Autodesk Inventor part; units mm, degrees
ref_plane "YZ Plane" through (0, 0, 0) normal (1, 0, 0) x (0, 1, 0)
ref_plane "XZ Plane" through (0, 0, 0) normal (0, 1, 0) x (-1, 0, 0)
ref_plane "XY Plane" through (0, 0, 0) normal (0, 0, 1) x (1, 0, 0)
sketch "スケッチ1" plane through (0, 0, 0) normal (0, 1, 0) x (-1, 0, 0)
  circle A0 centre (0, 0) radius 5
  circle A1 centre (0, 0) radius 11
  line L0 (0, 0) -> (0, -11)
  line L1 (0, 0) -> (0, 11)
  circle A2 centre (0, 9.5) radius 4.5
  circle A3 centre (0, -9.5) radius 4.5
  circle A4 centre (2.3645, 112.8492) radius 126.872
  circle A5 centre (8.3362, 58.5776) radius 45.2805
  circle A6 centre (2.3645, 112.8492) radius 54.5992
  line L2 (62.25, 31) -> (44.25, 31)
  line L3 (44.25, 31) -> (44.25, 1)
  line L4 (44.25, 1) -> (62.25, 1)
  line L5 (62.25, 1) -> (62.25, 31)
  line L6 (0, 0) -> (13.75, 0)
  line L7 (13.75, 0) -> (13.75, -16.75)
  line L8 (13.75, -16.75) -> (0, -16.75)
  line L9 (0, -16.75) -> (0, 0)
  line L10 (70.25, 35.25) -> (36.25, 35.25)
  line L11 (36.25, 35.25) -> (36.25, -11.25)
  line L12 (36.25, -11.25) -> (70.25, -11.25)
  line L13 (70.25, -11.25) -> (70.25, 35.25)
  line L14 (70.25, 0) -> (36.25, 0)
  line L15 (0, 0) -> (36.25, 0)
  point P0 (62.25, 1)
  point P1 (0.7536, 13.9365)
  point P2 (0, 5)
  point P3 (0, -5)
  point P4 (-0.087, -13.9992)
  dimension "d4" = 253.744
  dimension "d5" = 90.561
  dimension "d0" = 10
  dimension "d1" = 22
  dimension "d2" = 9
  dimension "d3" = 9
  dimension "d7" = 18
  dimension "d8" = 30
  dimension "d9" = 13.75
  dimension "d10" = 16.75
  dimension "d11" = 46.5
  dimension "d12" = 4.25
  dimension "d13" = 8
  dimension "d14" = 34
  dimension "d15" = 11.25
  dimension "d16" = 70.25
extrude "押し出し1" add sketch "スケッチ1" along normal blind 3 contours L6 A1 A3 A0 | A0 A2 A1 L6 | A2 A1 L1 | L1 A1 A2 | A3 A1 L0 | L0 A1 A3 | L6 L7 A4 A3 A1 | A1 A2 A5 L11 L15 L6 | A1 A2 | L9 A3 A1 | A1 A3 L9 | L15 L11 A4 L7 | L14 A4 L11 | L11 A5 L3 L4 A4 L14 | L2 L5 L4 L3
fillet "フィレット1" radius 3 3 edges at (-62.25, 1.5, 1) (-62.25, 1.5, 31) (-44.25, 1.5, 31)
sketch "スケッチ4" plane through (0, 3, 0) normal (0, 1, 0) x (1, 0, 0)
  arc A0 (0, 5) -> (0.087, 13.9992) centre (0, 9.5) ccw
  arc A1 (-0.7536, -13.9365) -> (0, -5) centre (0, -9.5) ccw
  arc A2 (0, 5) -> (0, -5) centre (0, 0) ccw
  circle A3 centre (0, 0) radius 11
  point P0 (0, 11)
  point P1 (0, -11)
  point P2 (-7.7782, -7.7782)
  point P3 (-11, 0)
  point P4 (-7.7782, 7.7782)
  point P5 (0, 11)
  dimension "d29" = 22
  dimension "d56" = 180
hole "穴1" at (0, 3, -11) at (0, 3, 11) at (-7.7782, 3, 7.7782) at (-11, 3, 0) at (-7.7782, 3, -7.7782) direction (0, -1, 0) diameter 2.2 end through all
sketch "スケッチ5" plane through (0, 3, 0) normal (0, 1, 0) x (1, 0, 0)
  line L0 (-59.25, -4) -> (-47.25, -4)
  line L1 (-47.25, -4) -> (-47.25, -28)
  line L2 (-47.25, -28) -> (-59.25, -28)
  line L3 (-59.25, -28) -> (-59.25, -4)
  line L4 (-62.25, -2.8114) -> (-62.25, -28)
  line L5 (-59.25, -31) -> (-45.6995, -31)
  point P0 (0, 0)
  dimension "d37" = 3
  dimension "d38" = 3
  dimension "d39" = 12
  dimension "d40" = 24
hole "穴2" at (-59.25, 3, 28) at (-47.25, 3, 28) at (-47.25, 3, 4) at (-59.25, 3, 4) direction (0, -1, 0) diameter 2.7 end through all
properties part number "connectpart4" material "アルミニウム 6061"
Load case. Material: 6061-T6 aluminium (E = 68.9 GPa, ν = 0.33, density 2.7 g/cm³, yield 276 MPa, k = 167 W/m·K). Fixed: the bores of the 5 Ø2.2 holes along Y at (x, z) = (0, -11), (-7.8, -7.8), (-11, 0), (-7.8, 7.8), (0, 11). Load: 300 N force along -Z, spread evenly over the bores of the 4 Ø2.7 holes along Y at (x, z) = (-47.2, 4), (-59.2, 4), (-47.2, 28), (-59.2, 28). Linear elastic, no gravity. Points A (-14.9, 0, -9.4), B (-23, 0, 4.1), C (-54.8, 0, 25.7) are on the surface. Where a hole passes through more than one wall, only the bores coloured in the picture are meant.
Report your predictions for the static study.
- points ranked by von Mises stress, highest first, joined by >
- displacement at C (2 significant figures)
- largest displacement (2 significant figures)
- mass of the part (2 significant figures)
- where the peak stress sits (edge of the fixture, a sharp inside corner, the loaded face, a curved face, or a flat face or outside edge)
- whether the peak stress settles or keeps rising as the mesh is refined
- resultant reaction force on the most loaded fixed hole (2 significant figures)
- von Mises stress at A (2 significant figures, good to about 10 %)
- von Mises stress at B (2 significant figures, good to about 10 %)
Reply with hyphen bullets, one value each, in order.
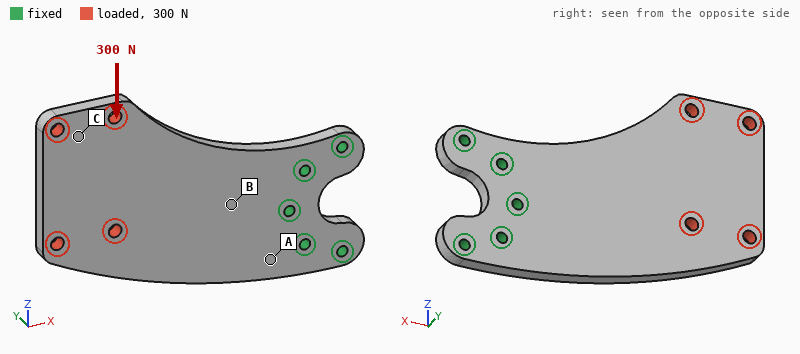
- A > B > C
- 46 µm
- 55 µm
- 15 g
- edge of the fixture
- keeps rising
- 530 N
- 24 MPa
- 10 MPa
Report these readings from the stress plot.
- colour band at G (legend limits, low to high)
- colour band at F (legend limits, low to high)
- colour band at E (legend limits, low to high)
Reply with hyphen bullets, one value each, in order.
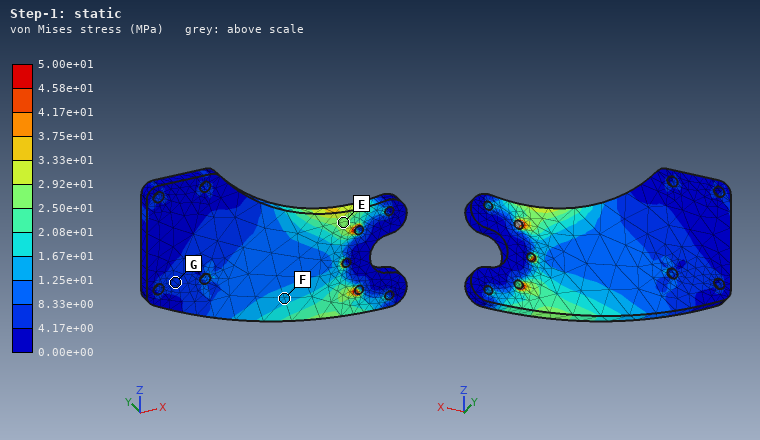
- 4.17e+00 to 8.33e+00 MPa
- 1.25e+01 to 1.67e+01 MPa
- 2.50e+01 to 2.92e+01 MPa
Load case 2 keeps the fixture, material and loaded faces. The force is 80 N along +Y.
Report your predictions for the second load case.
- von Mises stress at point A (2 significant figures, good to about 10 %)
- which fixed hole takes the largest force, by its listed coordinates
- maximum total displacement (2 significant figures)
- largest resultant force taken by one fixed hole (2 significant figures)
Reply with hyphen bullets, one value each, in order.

- 54 MPa
- (-11, 0)
- 0.84 mm
- 240 N
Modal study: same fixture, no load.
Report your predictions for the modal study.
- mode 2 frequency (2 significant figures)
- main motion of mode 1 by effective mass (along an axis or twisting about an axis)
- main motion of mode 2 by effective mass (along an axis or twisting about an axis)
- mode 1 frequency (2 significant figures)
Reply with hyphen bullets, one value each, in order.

- 2600 Hz
- along Y
- twisting about X
- 780 Hz
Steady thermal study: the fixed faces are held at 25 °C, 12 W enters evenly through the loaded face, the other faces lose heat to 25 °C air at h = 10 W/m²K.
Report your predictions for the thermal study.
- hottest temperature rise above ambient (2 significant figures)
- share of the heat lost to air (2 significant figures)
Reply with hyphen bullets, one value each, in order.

- 42 K
- 7.0 %
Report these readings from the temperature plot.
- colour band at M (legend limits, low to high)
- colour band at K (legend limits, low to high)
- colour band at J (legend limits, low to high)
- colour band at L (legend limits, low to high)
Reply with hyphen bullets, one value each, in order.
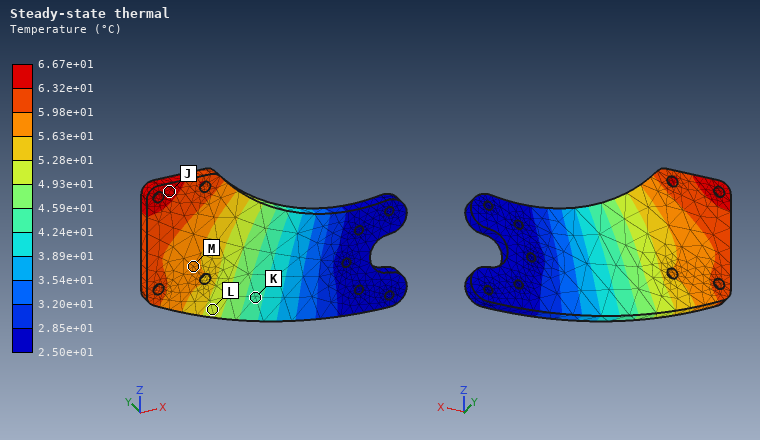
- 5.63e+01 to 5.98e+01 °C
- 4.24e+01 to 4.59e+01 °C
- 6.32e+01 to 6.67e+01 °C
- 4.93e+01 to 5.28e+01 °C
